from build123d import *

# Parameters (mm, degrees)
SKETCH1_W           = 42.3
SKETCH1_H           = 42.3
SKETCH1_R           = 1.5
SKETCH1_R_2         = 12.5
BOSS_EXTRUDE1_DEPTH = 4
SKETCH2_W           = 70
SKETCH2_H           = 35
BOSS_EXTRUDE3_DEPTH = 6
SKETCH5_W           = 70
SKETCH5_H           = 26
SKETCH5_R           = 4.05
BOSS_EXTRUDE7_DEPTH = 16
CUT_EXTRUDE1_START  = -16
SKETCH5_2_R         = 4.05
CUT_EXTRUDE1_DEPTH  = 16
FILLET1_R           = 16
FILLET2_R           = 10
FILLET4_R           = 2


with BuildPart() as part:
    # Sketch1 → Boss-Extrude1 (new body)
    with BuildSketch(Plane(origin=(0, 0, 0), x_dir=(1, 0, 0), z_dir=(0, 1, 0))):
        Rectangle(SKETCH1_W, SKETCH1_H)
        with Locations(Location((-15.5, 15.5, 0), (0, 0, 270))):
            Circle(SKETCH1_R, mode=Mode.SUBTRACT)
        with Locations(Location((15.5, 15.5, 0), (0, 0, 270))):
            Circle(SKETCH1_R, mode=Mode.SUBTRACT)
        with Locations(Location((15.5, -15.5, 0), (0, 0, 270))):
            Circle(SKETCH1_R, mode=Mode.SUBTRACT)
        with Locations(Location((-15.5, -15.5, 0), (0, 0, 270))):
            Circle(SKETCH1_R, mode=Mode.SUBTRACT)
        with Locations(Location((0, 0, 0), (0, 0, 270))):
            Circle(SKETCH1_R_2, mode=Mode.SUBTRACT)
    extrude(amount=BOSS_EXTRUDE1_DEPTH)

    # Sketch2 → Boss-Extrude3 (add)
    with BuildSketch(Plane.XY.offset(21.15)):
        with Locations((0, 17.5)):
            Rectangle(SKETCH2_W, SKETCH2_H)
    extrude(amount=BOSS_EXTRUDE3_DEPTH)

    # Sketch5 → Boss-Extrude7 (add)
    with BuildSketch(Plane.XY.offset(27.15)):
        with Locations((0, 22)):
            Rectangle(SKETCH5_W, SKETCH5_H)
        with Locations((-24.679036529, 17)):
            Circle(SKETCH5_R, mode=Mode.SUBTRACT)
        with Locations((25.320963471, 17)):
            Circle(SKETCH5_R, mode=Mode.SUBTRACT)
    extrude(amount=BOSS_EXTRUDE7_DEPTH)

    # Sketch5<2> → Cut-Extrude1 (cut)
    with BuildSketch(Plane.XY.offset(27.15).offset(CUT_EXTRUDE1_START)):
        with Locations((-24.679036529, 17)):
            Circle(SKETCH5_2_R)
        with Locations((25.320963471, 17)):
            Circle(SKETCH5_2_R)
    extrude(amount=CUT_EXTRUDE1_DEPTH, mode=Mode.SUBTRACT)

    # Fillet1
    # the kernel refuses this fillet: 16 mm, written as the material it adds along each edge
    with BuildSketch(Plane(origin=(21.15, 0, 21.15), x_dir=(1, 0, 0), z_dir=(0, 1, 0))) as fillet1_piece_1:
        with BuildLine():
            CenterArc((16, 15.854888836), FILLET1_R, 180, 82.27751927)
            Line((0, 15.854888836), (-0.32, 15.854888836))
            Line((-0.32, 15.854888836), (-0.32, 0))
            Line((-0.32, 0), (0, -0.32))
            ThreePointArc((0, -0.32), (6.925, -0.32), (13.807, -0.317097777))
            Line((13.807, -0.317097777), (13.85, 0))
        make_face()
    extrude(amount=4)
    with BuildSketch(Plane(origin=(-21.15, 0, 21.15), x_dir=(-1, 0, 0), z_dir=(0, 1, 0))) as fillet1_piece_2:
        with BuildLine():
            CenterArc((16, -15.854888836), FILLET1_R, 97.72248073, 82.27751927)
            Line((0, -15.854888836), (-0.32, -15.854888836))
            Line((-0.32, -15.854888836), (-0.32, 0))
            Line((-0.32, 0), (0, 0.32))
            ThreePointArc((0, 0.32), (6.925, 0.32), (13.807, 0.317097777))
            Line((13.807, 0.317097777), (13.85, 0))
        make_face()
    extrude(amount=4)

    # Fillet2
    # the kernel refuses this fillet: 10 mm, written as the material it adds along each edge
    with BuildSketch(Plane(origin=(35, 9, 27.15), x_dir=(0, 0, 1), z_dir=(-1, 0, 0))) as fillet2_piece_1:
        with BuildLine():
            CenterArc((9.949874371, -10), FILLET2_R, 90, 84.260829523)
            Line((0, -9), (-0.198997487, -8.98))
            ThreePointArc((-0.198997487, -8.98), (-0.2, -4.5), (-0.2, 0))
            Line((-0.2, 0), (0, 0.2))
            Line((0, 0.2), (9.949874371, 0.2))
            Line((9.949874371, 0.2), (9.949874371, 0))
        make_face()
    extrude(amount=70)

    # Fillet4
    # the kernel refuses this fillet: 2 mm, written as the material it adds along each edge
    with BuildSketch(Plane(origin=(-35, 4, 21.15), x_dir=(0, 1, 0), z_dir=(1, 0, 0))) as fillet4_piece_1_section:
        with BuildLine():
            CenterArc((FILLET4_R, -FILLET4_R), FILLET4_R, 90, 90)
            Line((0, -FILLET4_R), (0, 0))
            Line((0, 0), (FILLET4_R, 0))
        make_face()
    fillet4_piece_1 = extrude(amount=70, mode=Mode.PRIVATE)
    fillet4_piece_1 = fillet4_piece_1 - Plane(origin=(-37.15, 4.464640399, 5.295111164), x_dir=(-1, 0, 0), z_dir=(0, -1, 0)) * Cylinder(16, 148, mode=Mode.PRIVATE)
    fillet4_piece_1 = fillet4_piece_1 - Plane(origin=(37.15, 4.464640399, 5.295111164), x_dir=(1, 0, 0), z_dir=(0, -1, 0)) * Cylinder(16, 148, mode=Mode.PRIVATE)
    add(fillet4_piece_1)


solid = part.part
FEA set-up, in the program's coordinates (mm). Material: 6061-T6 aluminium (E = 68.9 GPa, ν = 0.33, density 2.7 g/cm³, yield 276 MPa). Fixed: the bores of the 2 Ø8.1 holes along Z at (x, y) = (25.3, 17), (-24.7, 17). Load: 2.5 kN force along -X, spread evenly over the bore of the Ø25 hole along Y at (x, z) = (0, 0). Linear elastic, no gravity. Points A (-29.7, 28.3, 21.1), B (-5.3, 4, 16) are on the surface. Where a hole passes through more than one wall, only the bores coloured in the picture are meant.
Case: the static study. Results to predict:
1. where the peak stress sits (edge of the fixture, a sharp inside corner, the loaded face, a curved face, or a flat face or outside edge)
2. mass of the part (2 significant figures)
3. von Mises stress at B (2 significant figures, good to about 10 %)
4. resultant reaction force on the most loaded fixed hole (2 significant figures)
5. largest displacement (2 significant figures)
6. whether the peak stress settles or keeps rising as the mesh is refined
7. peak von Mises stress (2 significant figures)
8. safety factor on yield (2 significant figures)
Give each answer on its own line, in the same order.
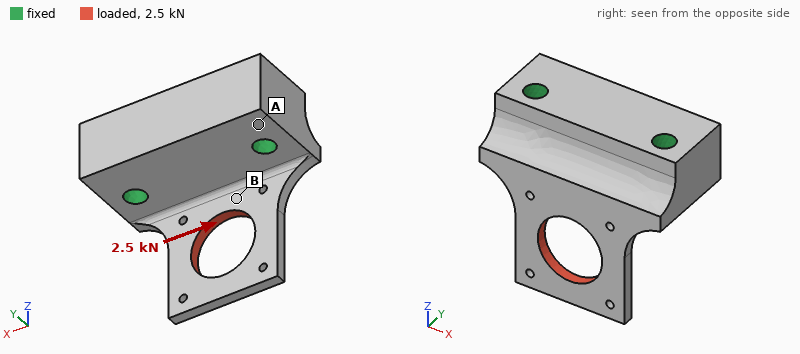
a curved face
130 g
41 MPa
2.0 kN
85 µm
settles
99 MPa
2.8
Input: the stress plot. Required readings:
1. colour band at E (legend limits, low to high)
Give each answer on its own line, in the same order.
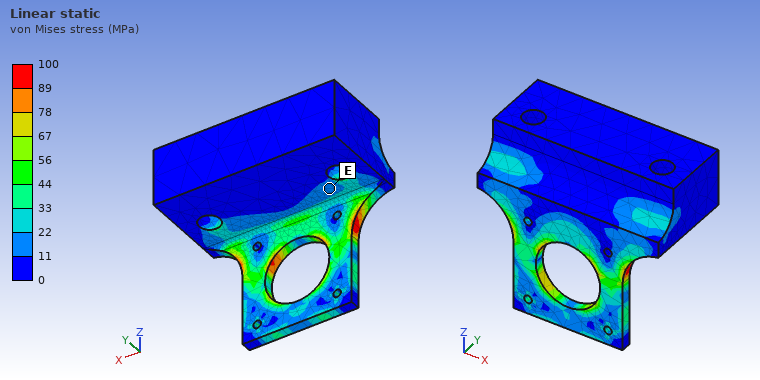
11 to 22 MPa
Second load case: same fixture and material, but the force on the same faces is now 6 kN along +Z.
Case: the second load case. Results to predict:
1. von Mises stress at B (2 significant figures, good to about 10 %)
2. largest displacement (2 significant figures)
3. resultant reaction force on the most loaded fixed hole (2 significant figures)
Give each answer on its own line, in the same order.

17 MPa
98 µm
3.1 kN
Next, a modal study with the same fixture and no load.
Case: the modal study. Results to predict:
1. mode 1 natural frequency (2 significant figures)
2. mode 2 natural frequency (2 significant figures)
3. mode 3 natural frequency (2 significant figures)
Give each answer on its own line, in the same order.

1600 Hz
3700 Hz
8200 Hz
